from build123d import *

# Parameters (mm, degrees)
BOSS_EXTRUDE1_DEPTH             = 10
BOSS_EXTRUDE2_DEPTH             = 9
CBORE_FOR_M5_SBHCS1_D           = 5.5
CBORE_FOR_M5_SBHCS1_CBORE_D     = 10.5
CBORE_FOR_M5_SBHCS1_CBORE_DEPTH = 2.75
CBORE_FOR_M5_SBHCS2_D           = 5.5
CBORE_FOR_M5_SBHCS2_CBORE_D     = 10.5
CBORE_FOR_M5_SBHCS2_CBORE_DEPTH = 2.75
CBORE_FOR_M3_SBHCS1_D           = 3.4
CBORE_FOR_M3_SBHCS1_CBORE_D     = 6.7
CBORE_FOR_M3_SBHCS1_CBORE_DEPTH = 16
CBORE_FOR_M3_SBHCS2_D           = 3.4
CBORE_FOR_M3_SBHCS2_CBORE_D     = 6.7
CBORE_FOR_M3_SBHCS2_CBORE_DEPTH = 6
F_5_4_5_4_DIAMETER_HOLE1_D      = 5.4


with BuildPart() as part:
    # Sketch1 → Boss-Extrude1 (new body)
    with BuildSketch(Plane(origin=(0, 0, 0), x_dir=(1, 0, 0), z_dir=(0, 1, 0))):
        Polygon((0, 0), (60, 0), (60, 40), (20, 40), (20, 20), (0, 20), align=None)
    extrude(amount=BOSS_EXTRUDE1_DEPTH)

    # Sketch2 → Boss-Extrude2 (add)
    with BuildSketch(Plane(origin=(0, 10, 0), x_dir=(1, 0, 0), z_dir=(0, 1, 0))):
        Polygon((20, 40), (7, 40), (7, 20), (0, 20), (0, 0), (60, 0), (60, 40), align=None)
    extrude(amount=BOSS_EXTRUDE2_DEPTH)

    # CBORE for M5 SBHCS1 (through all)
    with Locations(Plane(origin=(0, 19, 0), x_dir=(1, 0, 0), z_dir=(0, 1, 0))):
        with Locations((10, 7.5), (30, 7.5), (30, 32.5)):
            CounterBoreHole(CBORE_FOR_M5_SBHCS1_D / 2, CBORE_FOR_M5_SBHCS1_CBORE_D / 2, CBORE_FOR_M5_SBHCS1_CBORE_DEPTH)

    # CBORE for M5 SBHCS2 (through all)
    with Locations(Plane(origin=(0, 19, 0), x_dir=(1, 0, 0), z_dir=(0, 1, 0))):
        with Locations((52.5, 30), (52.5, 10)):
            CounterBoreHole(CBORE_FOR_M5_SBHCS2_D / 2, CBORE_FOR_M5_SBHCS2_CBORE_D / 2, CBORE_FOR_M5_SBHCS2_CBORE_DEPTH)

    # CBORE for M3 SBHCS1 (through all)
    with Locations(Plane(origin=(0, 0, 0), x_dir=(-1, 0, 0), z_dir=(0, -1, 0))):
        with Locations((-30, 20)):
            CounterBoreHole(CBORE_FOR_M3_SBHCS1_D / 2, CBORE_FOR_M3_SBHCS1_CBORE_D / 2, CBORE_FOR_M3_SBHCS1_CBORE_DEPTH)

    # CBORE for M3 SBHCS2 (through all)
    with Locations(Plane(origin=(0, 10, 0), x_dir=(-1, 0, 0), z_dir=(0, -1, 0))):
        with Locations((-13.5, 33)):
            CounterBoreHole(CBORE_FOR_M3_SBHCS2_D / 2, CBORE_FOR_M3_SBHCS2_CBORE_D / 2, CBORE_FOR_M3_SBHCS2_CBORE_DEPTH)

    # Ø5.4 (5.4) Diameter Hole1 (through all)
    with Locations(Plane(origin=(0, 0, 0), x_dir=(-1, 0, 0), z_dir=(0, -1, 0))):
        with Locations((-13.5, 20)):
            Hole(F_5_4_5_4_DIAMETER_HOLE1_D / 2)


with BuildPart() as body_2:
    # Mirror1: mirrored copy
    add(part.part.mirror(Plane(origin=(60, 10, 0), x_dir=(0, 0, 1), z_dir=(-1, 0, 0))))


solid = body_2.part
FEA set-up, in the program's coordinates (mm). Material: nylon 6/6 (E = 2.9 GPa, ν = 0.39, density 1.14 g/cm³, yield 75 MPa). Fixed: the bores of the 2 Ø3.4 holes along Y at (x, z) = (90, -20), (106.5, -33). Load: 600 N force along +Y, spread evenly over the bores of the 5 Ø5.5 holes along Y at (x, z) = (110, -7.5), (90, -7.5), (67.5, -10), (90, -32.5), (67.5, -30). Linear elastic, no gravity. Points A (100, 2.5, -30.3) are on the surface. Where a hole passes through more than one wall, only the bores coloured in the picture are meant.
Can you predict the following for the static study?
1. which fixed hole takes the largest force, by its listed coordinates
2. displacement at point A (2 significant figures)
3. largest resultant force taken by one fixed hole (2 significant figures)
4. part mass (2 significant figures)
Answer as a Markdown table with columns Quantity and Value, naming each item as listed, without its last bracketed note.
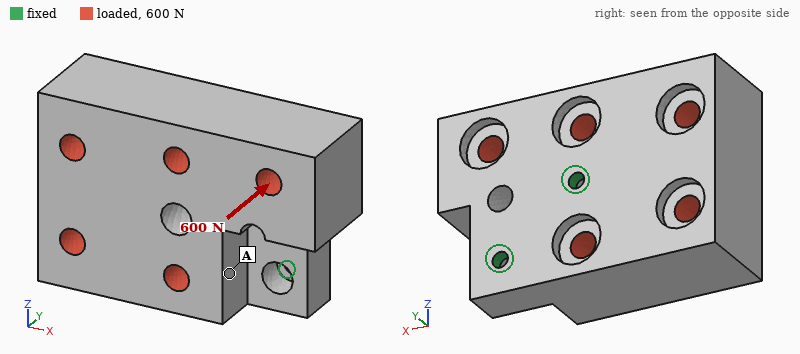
| Quantity | Value |
|---|---|
| which fixed hole takes the largest force, by its listed coordinates | (90, -20) |
| displacement at point A | 0.092 mm |
| largest resultant force taken by one fixed hole | 730 N |
| part mass | 41 g |
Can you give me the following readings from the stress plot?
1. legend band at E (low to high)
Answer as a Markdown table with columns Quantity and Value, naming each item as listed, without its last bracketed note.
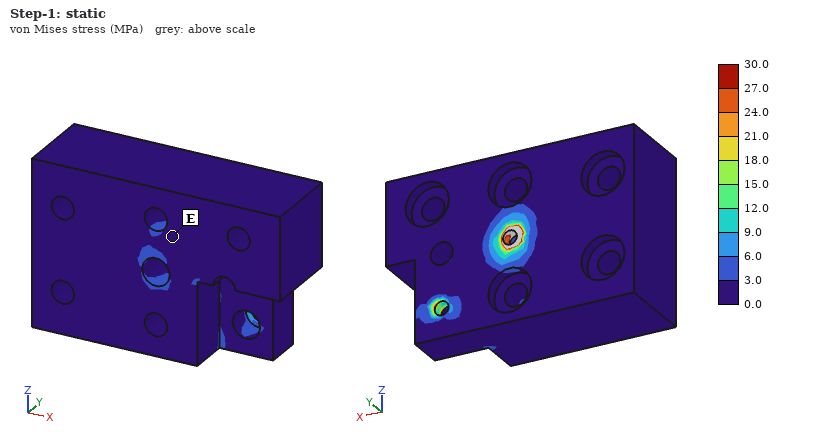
| Quantity | Value |
|---|---|
| legend band at E | 0.0 to 3.0 MPa |
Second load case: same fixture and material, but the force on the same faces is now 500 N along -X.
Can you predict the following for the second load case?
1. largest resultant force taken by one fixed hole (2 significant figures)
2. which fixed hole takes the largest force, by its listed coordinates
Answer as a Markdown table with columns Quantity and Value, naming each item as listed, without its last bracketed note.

| Quantity | Value |
|---|---|
| largest resultant force taken by one fixed hole | 440 N |
| which fixed hole takes the largest force, by its listed coordinates | (90, -20) |
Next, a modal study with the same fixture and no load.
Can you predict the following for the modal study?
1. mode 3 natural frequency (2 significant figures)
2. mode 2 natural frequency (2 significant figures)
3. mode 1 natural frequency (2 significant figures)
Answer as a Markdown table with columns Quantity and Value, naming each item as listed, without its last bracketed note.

| Quantity | Value |
|---|---|
| mode 3 natural frequency | 1900 Hz |
| mode 2 natural frequency | 1600 Hz |
| mode 1 natural frequency | 560 Hz |
